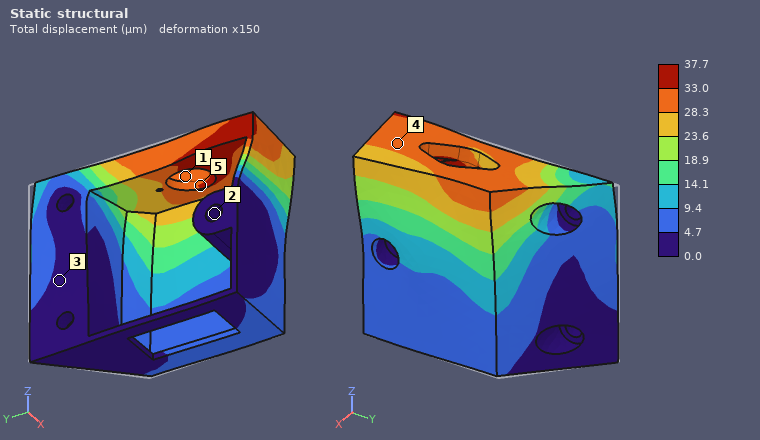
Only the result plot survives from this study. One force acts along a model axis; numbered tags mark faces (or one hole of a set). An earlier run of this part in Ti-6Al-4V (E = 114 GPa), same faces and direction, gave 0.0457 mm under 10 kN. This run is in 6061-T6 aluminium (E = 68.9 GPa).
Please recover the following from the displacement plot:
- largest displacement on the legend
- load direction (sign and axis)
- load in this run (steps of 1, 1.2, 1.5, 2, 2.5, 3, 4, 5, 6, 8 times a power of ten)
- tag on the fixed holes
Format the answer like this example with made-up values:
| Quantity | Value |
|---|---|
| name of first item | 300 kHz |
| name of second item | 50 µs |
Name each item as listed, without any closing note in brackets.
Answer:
| Quantity | Value |
|---|---|
| largest displacement on the legend | 37.7 µm |
| load direction | -Y |
| load in this run | 5 kN |
| tag on the fixed holes | 2 |
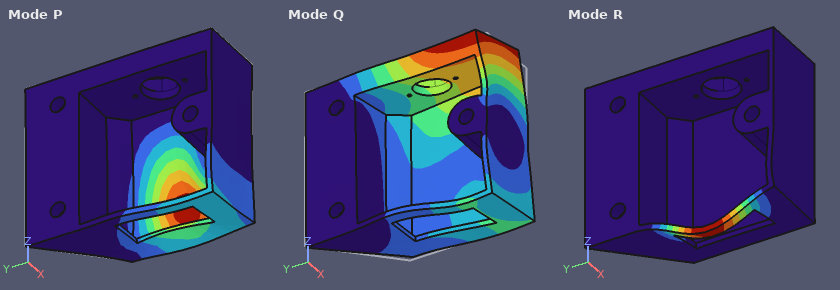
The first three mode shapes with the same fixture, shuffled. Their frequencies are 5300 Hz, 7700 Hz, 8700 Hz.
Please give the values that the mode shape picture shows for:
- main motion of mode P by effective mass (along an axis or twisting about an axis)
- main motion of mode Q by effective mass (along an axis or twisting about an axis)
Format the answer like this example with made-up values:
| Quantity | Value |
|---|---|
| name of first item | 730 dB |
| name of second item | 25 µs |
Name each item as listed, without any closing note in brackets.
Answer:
| Quantity | Value |
|---|---|
| main motion of mode P by effective mass | along X |
| main motion of mode Q by effective mass | along X |
